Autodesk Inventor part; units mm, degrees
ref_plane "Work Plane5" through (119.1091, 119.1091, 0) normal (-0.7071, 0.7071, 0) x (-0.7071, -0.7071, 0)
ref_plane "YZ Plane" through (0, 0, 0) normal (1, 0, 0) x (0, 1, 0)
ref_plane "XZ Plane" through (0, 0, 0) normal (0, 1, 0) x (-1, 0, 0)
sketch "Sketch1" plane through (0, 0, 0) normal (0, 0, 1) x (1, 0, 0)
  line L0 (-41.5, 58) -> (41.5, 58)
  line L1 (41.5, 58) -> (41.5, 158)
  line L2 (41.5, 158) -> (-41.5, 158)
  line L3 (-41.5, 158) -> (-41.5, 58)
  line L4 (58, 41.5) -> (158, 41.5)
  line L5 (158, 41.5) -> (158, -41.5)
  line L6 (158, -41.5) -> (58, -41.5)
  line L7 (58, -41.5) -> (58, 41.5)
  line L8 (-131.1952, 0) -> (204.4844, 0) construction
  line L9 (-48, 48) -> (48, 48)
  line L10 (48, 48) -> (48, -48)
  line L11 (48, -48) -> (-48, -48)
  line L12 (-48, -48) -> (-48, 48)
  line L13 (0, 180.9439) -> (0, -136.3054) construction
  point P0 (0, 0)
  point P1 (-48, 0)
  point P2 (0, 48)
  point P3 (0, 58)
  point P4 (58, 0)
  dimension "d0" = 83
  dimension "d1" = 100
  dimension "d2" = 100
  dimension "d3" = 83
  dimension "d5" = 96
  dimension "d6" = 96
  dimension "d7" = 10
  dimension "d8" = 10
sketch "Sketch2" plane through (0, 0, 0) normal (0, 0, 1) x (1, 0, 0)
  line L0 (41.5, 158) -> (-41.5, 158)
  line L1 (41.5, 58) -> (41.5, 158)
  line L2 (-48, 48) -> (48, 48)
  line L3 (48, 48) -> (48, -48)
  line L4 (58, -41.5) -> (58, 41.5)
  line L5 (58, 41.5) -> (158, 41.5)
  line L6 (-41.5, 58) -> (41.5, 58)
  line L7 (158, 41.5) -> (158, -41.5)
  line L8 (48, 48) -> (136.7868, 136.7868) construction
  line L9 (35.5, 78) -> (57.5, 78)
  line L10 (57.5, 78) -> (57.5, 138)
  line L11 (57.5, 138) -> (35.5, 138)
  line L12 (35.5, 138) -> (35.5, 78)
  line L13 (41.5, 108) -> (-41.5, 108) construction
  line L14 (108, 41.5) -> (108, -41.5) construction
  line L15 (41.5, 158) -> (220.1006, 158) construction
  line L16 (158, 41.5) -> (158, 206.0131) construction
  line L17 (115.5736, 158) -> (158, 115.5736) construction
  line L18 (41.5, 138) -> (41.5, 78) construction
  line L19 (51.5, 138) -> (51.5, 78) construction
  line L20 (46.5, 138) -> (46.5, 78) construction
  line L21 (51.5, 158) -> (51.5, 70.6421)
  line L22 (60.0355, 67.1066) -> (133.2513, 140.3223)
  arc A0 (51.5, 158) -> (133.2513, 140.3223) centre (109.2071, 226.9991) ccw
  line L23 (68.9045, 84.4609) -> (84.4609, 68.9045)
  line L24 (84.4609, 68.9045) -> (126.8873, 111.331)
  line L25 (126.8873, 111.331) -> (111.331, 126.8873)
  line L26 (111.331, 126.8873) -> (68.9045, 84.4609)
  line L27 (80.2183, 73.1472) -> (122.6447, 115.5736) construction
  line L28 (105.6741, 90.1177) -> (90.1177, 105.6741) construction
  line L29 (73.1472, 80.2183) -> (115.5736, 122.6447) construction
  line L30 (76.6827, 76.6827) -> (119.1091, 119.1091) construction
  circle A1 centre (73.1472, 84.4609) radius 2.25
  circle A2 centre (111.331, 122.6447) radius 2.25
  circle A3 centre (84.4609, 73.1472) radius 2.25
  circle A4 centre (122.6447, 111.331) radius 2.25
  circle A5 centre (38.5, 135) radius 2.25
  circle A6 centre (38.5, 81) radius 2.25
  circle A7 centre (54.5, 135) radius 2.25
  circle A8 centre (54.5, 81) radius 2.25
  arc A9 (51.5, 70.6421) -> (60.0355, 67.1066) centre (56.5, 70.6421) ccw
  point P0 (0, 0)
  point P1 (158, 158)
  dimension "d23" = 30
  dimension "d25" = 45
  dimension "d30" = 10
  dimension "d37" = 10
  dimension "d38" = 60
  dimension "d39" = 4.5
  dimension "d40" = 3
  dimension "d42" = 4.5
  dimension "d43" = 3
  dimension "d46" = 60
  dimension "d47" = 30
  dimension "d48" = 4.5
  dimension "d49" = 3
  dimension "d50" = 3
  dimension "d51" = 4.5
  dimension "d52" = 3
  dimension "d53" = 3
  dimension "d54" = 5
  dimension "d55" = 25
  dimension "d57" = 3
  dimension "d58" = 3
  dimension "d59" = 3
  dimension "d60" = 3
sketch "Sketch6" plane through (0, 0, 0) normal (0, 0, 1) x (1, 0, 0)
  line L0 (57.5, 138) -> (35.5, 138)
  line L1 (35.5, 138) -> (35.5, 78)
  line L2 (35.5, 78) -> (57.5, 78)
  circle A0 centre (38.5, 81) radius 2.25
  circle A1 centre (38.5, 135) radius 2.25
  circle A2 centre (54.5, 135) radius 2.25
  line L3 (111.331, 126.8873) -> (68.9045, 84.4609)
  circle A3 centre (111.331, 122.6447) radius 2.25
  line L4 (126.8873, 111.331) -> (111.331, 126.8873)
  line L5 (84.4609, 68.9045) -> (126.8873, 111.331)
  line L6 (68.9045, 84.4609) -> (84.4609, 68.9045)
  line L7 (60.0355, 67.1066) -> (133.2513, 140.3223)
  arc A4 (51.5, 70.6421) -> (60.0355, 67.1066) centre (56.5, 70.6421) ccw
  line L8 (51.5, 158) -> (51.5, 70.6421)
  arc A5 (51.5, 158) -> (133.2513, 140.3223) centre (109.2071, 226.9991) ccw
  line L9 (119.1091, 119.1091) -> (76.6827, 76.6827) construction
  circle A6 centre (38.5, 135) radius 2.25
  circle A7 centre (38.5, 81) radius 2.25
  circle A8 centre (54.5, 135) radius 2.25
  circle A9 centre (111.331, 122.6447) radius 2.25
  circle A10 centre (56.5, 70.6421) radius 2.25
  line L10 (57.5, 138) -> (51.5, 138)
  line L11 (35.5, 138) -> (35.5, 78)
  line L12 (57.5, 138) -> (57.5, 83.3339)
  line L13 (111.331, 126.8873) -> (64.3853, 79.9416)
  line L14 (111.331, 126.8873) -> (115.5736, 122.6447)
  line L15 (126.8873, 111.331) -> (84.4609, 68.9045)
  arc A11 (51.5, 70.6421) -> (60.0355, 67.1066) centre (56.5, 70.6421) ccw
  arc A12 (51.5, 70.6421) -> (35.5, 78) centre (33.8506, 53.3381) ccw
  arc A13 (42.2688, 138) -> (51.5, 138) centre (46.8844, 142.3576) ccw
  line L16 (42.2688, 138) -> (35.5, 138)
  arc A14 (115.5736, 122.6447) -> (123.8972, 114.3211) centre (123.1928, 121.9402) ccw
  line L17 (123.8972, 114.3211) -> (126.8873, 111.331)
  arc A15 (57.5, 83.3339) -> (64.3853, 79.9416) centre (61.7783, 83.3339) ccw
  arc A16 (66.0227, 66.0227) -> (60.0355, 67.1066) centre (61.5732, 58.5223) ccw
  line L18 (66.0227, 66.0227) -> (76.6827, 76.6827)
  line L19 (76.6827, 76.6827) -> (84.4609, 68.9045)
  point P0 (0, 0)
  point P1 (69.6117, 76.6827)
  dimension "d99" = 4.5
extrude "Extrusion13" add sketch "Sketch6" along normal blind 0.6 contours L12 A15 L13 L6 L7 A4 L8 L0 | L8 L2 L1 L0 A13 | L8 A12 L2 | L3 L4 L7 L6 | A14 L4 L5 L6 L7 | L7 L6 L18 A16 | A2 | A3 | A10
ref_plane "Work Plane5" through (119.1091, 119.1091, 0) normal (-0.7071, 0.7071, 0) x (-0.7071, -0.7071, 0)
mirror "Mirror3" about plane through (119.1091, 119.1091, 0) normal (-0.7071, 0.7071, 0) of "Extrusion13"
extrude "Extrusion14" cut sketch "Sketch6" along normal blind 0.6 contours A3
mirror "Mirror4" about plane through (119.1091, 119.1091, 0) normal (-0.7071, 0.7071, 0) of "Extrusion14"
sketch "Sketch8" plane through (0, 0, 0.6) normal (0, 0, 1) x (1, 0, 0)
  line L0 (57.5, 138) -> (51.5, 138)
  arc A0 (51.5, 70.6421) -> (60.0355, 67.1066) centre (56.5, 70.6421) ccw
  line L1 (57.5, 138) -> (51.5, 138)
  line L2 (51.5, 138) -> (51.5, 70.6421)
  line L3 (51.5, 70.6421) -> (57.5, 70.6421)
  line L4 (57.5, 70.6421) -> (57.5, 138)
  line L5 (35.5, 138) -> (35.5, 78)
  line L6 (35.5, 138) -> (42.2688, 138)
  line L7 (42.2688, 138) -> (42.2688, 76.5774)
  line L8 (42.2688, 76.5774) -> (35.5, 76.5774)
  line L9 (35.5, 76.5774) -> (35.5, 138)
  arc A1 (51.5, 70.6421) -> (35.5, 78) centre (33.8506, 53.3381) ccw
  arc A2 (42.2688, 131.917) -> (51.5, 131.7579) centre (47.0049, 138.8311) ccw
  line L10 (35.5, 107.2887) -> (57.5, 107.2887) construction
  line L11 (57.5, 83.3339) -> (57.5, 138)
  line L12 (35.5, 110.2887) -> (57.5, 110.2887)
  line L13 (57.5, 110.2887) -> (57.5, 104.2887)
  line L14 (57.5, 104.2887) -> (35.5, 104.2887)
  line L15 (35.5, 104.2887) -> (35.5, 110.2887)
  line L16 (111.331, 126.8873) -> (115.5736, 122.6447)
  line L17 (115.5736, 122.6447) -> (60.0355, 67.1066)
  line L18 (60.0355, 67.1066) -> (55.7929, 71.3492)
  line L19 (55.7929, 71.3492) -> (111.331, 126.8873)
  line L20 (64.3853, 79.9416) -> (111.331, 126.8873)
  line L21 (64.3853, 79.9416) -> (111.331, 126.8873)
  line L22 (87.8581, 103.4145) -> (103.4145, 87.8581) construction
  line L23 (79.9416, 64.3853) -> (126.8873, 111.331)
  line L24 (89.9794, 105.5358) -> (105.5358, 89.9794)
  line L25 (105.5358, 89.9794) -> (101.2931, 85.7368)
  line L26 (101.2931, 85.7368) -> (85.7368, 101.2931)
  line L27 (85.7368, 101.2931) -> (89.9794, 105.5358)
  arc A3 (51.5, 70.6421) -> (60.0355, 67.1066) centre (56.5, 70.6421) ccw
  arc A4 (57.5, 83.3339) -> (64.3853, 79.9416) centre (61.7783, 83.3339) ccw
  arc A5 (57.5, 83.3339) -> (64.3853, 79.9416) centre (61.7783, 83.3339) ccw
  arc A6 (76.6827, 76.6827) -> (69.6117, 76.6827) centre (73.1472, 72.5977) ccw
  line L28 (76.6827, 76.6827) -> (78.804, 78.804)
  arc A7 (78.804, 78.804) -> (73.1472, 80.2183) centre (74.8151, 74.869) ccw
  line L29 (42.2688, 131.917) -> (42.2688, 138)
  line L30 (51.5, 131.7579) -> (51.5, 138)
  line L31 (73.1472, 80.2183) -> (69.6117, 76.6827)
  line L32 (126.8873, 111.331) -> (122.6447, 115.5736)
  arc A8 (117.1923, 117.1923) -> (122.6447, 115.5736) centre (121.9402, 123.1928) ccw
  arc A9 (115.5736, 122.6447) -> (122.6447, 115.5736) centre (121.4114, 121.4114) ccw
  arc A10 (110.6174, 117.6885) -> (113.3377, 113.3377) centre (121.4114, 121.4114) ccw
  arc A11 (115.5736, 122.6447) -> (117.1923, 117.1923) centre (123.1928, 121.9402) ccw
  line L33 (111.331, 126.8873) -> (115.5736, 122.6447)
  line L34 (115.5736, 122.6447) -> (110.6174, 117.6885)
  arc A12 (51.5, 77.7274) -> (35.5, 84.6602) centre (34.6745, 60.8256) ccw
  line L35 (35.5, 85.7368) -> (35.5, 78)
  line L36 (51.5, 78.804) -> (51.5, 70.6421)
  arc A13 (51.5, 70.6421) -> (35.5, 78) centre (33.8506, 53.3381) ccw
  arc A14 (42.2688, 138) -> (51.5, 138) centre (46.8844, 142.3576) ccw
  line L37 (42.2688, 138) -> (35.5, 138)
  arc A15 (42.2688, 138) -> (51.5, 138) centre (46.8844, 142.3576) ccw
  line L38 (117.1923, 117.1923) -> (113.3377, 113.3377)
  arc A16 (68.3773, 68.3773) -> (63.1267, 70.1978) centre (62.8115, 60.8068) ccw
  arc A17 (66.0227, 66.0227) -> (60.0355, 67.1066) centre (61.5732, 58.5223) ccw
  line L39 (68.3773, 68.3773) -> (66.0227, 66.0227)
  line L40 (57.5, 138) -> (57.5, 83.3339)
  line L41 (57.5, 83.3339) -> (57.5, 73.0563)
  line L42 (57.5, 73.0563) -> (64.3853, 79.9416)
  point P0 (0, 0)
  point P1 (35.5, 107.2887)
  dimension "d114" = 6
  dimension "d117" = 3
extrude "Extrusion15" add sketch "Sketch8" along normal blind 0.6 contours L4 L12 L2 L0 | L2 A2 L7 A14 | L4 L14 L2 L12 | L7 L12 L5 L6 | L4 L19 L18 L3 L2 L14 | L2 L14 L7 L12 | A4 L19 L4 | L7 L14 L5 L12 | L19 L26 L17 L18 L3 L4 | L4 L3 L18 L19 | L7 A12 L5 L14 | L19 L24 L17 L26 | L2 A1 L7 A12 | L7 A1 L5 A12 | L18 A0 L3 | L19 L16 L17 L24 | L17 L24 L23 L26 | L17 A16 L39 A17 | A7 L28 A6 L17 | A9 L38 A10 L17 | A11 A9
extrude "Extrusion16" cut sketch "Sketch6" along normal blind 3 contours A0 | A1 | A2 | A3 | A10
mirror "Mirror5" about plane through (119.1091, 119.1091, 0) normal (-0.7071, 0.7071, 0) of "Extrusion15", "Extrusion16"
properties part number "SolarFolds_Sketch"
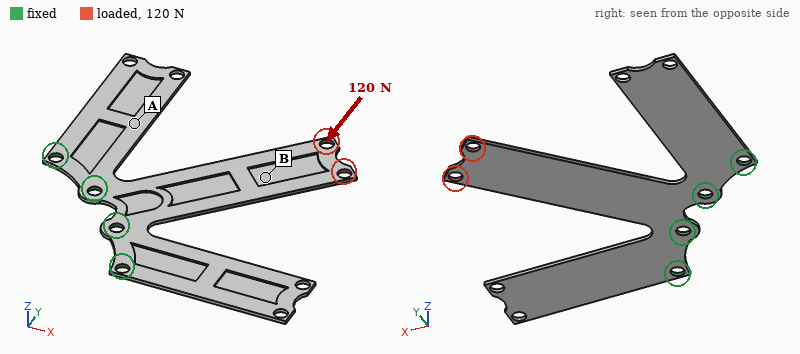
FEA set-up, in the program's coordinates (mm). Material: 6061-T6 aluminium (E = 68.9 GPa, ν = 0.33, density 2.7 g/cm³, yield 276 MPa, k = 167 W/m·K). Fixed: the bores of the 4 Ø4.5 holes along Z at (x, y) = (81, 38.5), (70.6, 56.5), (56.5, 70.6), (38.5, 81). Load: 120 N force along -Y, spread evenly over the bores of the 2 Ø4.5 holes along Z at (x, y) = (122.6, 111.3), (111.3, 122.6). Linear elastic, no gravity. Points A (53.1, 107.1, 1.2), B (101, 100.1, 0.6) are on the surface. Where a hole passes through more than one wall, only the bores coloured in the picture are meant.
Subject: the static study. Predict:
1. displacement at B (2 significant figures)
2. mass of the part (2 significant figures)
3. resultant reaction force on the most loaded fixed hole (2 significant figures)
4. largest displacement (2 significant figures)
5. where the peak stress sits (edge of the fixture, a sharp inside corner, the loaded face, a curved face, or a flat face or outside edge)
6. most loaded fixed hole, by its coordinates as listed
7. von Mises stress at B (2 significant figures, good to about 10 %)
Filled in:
0.092 mm
12 g
310 N
0.25 mm
a curved face
(70.6, 56.5)
20 MPa
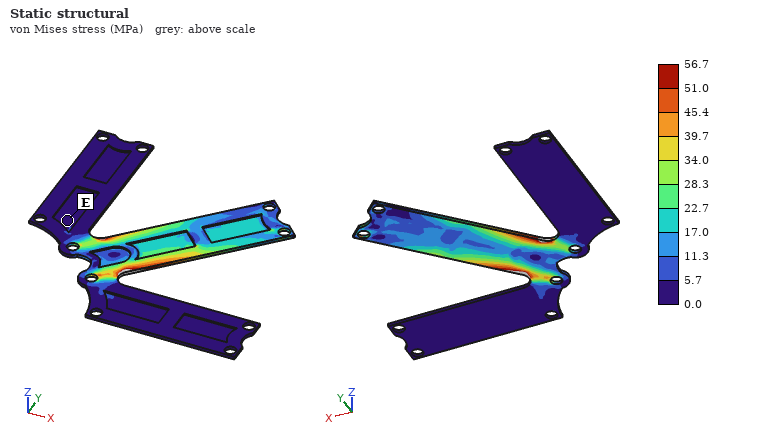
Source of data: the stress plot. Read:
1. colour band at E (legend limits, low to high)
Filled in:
0.0 to 5.7 MPa
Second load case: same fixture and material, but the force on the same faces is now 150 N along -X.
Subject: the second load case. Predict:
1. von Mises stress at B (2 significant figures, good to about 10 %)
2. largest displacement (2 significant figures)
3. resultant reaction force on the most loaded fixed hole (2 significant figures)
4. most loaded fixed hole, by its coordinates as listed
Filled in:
24 MPa
0.32 mm
390 N
(56.5, 70.6)
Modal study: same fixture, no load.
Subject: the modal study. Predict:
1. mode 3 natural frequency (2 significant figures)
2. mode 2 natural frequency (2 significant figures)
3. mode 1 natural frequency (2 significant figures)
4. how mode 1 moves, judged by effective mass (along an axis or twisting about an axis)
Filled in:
300 Hz
300 Hz
170 Hz
along Z
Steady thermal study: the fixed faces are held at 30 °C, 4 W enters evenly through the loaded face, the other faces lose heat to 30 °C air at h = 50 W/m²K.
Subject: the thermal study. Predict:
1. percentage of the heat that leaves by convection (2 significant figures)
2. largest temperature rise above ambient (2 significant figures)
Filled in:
73 %
46 K
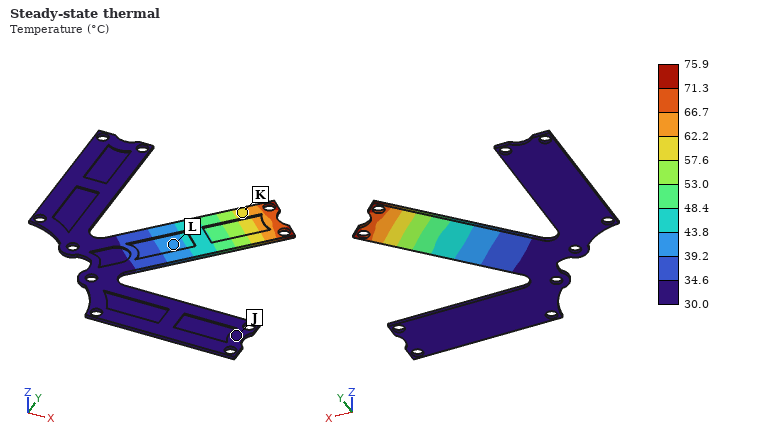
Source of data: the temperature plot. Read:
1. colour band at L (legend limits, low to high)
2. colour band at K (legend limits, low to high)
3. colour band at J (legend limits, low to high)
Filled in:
39.2 to 43.8 °C
57.6 to 62.2 °C
30.0 to 34.6 °C
